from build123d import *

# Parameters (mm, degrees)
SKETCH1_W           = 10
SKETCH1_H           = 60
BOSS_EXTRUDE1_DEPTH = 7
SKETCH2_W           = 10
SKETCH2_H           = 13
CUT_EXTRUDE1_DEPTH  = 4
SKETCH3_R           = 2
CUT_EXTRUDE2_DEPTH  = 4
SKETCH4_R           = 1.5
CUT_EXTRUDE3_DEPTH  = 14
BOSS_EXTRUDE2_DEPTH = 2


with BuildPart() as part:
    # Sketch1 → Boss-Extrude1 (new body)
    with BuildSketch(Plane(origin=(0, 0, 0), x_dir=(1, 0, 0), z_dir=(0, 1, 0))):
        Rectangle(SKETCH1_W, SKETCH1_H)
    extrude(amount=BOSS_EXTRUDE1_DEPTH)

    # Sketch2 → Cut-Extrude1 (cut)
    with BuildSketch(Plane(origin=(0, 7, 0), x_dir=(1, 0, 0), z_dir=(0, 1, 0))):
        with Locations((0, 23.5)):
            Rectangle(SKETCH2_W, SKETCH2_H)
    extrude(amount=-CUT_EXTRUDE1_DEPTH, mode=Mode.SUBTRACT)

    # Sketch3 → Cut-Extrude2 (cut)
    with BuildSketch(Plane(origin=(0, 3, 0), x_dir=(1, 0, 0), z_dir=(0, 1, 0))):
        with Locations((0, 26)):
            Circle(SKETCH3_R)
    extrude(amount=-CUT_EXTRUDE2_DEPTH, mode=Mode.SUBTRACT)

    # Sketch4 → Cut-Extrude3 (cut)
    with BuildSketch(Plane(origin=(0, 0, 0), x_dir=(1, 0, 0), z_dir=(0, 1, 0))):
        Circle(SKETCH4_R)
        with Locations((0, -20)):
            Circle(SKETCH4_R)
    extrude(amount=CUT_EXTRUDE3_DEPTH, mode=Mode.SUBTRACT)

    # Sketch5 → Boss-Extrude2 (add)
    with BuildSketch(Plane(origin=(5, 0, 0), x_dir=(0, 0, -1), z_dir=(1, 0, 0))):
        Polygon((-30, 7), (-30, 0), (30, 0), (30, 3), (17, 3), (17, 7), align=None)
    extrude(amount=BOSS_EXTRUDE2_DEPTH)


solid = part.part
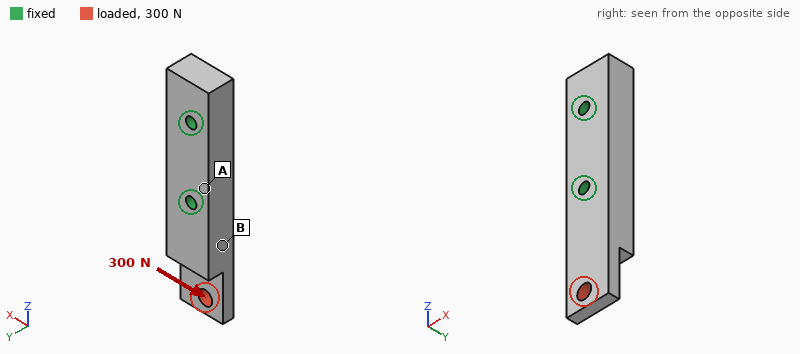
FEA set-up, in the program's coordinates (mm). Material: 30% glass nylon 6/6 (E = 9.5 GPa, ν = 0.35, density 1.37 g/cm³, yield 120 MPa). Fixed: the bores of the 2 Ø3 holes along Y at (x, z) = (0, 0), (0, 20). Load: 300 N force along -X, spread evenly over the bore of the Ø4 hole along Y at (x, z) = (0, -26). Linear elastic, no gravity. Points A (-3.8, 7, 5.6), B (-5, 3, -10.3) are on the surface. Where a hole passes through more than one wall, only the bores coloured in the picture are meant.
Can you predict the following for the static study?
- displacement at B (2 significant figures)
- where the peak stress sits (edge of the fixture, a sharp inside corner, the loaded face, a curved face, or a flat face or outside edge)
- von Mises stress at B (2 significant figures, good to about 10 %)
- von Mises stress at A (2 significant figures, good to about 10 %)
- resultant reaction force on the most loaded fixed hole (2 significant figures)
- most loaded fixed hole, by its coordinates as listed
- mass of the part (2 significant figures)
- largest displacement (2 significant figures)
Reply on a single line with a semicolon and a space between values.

0.11 mm; edge of the fixture; 31 MPa; 13 MPa; 570 N; (0, 0); 5.9 g; 0.46 mm
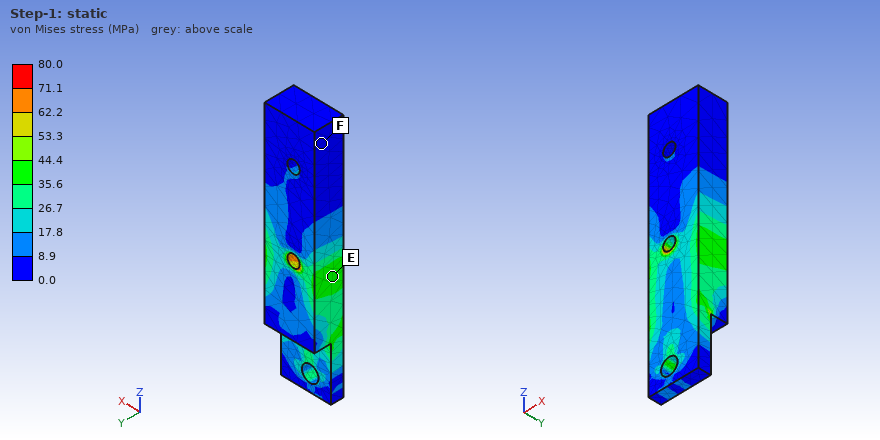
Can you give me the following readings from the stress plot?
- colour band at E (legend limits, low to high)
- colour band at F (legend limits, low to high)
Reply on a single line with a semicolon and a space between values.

35.6 to 44.4 MPa; 0.0 to 8.9 MPa
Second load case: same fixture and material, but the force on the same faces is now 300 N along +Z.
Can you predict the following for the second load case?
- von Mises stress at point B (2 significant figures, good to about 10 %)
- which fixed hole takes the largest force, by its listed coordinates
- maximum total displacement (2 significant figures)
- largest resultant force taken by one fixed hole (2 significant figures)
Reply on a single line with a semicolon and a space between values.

6.3 MPa; (0, 0); 82 µm; 270 N
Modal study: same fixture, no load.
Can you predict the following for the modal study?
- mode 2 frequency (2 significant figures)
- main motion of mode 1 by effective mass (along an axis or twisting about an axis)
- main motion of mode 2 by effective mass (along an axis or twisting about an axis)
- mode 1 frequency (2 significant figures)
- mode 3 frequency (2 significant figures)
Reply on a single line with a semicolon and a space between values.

5800 Hz; along Y; along X; 4000 Hz; 11 kHz
